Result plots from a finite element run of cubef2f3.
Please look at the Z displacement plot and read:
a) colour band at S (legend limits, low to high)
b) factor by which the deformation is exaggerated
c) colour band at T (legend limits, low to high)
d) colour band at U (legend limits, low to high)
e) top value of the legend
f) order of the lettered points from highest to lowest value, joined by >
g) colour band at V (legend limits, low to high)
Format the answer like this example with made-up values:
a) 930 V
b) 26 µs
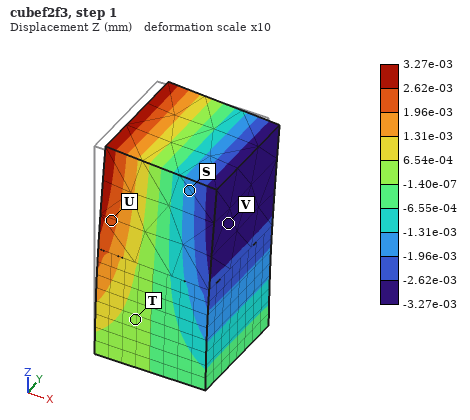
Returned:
a) -1.96e-03 to -1.31e-03 mm
b) 10
c) -1.40e-07 to 6.54e-04 mm
d) 1.96e-03 to 2.62e-03 mm
e) 3.27e-03 mm
f) U > T > S > V
g) -3.27e-03 to -2.62e-03 mm
